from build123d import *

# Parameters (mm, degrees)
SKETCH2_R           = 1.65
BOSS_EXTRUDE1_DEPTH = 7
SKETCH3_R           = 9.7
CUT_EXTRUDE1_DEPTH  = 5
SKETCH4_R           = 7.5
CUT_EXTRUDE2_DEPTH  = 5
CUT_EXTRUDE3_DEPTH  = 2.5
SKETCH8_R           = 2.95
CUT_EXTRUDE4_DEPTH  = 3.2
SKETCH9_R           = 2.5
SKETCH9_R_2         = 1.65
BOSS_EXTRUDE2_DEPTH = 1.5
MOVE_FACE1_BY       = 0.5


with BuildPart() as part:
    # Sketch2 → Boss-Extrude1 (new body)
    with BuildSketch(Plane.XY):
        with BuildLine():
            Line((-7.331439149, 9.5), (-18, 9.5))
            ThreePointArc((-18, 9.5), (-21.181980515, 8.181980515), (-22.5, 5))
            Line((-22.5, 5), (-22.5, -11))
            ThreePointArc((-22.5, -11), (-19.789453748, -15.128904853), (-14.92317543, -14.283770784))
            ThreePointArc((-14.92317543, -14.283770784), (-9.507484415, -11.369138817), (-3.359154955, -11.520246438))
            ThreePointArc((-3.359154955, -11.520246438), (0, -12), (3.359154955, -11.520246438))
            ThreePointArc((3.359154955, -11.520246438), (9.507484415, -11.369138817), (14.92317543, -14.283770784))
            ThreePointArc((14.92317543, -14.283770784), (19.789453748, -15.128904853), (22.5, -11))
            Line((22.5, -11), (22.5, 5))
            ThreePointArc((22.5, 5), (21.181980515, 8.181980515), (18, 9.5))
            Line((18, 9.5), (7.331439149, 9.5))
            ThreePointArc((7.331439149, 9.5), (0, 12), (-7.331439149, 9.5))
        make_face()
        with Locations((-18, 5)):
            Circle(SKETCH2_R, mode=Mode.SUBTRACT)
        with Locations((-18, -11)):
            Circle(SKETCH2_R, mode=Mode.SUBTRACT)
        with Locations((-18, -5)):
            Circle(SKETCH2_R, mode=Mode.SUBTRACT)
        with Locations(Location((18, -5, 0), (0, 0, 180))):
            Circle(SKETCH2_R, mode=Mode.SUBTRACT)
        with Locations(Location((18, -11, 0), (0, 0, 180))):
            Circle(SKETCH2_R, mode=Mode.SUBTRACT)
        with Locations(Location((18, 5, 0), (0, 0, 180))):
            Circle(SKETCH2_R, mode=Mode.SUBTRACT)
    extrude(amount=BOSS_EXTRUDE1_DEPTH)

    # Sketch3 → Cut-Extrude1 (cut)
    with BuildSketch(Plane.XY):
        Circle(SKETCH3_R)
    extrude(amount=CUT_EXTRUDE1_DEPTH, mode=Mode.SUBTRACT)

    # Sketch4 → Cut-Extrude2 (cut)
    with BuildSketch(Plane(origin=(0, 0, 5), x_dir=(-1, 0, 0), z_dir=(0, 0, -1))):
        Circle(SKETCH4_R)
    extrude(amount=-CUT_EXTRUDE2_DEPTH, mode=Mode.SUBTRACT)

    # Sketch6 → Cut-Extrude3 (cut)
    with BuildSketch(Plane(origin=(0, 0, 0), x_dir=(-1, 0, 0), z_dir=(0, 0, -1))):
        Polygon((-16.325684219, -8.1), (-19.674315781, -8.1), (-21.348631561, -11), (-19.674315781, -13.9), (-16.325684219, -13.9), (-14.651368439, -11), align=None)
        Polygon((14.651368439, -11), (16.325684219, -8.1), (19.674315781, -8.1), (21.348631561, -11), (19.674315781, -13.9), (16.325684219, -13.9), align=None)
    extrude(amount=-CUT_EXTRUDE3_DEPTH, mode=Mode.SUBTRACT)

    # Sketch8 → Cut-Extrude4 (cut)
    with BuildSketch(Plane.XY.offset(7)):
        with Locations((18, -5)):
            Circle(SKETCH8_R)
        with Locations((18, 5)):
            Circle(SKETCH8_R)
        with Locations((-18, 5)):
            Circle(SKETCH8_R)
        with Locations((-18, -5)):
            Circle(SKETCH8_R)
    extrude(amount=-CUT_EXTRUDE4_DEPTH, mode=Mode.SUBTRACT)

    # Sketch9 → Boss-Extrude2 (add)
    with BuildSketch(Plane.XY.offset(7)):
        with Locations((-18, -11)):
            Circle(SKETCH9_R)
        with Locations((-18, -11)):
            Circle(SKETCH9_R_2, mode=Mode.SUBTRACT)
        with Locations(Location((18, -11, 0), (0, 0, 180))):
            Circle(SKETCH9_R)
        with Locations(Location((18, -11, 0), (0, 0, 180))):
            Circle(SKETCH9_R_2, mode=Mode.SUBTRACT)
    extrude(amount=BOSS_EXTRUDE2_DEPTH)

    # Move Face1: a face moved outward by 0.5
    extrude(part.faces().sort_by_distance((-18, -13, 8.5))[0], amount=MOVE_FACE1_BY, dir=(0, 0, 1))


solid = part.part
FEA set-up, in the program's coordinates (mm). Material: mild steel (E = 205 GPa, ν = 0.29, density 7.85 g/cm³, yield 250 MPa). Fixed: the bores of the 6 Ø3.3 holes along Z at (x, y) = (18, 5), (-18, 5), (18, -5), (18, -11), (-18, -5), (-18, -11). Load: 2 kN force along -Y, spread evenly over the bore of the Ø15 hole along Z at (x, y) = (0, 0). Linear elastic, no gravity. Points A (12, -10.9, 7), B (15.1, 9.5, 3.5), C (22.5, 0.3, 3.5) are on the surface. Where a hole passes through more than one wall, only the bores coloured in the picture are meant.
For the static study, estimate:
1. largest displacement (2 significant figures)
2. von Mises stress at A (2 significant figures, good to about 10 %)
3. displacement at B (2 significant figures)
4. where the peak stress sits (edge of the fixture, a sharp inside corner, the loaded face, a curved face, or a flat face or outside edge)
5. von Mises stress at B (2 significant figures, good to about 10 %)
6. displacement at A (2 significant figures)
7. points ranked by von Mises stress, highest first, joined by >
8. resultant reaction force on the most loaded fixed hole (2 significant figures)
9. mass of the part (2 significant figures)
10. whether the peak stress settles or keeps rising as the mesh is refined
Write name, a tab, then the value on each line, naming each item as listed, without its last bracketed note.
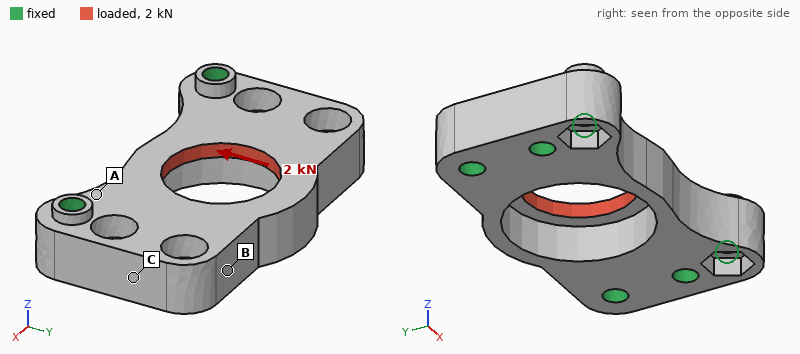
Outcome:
largest displacement	5.7 µm
von Mises stress at A	18 MPa
displacement at B	0.86 µm
where the peak stress sits	edge of the fixture
von Mises stress at B	13 MPa
displacement at A	0.90 µm
points ranked by von Mises stress, highest first, joined by >	A > B > C
resultant reaction force on the most loaded fixed hole	550 N
mass of the part	36 g
whether the peak stress settles or keeps rising as the mesh is refined	keeps rising
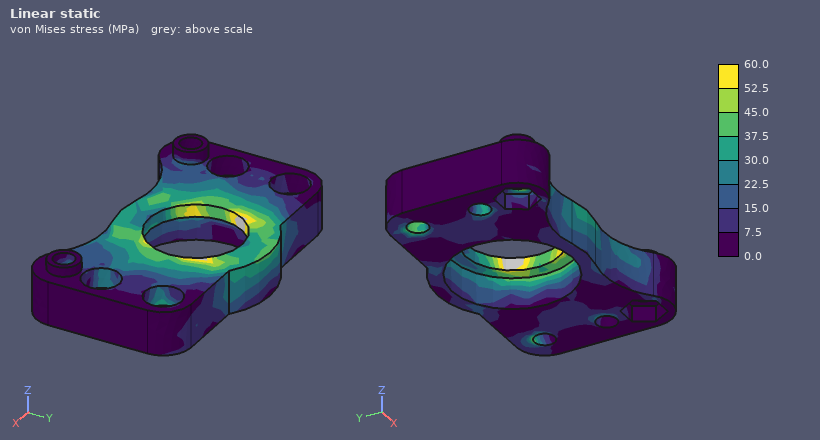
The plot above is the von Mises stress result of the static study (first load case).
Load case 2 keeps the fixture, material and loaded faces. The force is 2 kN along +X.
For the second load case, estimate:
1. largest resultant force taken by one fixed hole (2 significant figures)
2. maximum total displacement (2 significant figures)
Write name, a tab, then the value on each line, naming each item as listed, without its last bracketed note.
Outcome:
largest resultant force taken by one fixed hole	540 N
maximum total displacement	2.0 µm
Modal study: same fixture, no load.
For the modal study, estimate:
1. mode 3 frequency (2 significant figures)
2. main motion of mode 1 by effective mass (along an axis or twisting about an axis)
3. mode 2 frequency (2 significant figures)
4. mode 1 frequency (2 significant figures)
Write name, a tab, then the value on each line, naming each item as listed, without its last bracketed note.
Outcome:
mode 3 frequency	41 kHz
main motion of mode 1 by effective mass	along Z
mode 2 frequency	29 kHz
mode 1 frequency	23 kHz
